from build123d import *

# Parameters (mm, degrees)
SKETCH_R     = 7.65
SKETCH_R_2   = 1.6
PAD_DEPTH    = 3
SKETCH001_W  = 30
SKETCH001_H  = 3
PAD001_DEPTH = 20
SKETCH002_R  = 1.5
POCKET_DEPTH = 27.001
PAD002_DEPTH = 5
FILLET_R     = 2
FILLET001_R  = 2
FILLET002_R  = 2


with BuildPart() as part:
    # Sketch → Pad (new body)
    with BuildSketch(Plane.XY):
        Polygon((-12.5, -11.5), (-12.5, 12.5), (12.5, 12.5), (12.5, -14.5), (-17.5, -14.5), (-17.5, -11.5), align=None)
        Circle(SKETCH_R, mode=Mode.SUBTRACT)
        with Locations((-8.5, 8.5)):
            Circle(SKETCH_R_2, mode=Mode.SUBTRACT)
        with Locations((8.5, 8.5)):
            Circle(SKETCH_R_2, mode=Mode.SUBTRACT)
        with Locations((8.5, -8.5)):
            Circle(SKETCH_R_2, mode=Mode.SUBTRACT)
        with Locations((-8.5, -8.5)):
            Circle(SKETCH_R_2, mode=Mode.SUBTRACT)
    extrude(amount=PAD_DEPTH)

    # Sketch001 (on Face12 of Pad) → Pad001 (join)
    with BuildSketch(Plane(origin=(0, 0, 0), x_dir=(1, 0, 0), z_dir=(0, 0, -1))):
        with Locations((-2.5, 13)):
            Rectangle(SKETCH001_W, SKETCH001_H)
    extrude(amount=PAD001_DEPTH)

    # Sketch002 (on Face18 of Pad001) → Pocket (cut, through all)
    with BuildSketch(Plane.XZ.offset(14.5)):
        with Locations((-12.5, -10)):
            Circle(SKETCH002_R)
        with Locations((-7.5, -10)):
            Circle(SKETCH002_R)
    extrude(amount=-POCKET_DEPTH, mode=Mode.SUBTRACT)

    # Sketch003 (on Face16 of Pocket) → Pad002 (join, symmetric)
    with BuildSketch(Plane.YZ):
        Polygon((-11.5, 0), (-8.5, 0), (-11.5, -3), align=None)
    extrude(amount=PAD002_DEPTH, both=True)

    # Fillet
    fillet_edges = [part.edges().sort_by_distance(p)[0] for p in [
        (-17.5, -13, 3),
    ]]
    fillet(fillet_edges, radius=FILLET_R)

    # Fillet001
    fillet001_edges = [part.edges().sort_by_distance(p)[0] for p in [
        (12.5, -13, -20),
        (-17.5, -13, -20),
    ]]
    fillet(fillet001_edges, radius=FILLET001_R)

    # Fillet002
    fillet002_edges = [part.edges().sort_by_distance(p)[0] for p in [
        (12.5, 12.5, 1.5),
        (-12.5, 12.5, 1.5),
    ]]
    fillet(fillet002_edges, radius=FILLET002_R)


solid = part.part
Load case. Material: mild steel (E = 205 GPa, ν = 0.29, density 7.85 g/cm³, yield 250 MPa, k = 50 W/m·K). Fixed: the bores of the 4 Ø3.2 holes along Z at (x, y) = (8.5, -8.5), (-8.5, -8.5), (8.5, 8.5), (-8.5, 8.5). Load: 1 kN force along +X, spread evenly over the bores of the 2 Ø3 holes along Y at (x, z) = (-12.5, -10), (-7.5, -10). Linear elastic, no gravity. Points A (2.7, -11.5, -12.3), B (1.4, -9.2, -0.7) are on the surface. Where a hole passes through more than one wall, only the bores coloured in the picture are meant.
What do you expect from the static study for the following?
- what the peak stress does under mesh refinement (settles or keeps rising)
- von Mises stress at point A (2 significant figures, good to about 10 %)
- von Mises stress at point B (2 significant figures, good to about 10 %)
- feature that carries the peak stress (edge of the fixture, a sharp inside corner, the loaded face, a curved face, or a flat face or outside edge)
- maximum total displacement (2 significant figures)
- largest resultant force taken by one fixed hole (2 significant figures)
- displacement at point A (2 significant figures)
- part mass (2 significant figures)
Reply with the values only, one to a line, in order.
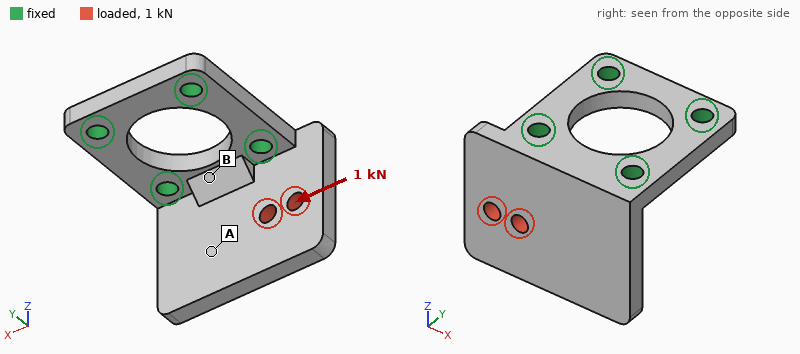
keeps rising
17 MPa
45 MPa
edge of the fixture
13 µm
840 N
7.0 µm
25 g
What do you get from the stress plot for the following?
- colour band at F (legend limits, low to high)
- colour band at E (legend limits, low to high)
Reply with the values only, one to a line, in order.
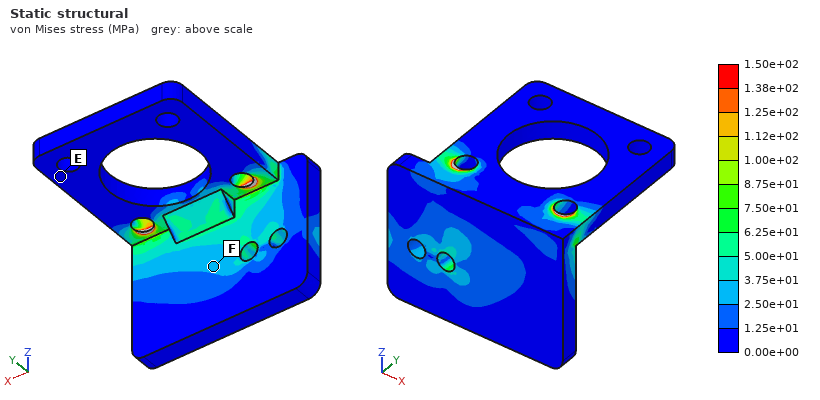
2.50e+01 to 3.75e+01 MPa
0.00e+00 to 1.25e+01 MPa
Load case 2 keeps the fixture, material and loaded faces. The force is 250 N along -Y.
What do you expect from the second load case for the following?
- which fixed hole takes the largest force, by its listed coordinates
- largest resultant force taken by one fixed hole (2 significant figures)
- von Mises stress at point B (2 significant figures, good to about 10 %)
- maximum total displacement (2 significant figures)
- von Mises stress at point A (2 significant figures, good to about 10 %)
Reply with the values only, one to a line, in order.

(-8.5, -8.5)
250 N
34 MPa
48 µm
19 MPa
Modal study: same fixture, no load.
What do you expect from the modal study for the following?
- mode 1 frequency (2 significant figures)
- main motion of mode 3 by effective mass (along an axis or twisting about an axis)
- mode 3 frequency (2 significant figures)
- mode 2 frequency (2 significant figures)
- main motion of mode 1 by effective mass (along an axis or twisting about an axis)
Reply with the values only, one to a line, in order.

4400 Hz
along X
15 kHz
8700 Hz
along Y
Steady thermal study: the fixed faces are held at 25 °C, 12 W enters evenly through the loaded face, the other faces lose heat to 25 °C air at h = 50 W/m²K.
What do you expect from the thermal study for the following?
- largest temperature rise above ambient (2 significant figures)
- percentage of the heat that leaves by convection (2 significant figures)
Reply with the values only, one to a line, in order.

57 K
19 %
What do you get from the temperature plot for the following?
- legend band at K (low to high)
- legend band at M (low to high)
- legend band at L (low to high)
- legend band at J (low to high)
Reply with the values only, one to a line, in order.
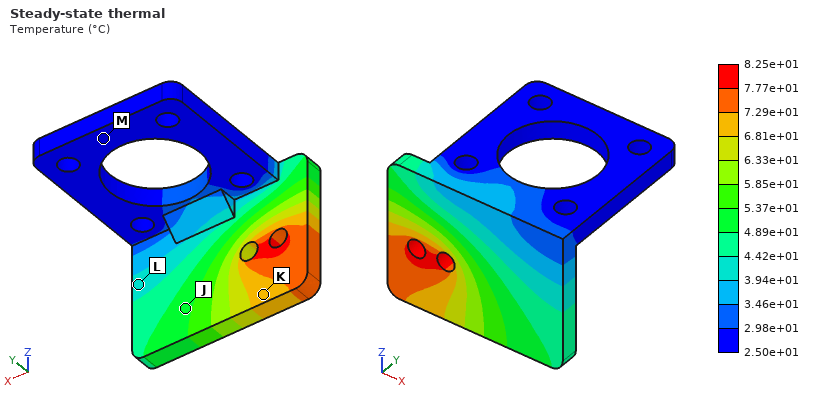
6.81e+01 to 7.29e+01 °C
2.50e+01 to 2.98e+01 °C
3.94e+01 to 4.42e+01 °C
4.89e+01 to 5.37e+01 °C
